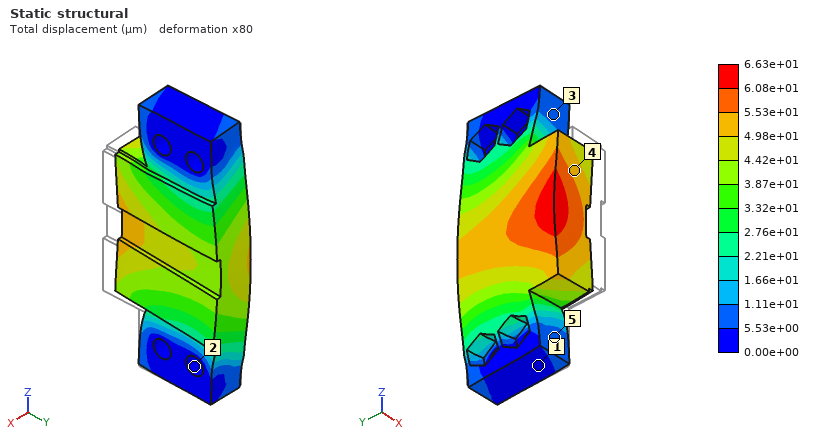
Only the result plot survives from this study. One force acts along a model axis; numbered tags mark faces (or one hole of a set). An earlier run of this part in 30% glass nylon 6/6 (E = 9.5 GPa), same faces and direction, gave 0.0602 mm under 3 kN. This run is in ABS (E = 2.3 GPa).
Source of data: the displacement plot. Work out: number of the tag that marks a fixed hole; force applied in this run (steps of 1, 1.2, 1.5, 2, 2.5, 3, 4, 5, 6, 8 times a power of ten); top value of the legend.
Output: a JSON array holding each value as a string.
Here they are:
["2", "800 N", "6.63e+01 µm"]
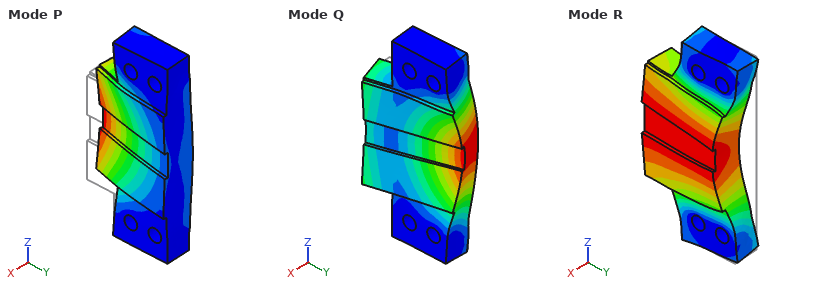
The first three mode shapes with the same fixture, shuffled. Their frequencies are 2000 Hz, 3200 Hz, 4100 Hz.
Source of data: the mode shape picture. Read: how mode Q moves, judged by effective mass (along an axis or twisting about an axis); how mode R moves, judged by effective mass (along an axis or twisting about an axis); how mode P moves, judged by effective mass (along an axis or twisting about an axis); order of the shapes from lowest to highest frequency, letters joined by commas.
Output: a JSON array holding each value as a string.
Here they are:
["along X", "along Y", "along X", "P, Q, R"]
